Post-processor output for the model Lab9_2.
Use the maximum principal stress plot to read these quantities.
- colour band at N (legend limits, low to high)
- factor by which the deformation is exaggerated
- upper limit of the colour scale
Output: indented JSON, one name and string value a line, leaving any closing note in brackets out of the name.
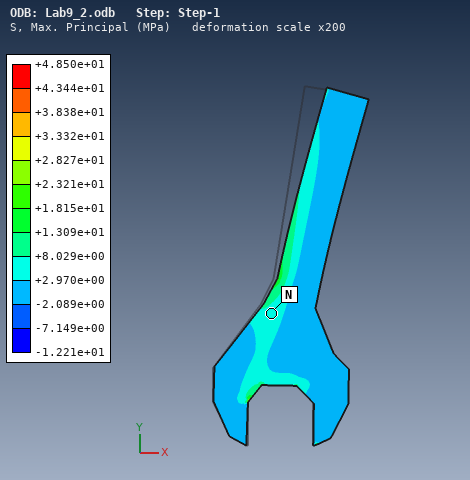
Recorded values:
{
  "colour band at N": "+2.970e+00 to +8.029e+00 MPa",
  "factor by which the deformation is exaggerated": "200",
  "upper limit of the colour scale": "+4.850e+01 MPa"
}
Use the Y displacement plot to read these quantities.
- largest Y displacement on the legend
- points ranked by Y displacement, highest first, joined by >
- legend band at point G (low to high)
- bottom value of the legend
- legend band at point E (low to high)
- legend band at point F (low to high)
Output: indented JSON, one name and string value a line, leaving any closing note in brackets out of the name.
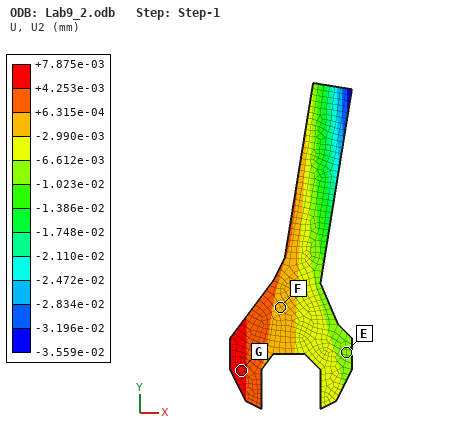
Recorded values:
{
  "largest Y displacement on the legend": "+7.875e-03 mm",
  "points ranked by Y displacement, highest first, joined by >": "G > F > E",
  "legend band at point G": "+4.253e-03 to +7.875e-03 mm",
  "bottom value of the legend": "-3.559e-02 mm",
  "legend band at point E": "-1.023e-02 to -6.612e-03 mm",
  "legend band at point F": "-2.990e-03 to +6.315e-04 mm"
}
